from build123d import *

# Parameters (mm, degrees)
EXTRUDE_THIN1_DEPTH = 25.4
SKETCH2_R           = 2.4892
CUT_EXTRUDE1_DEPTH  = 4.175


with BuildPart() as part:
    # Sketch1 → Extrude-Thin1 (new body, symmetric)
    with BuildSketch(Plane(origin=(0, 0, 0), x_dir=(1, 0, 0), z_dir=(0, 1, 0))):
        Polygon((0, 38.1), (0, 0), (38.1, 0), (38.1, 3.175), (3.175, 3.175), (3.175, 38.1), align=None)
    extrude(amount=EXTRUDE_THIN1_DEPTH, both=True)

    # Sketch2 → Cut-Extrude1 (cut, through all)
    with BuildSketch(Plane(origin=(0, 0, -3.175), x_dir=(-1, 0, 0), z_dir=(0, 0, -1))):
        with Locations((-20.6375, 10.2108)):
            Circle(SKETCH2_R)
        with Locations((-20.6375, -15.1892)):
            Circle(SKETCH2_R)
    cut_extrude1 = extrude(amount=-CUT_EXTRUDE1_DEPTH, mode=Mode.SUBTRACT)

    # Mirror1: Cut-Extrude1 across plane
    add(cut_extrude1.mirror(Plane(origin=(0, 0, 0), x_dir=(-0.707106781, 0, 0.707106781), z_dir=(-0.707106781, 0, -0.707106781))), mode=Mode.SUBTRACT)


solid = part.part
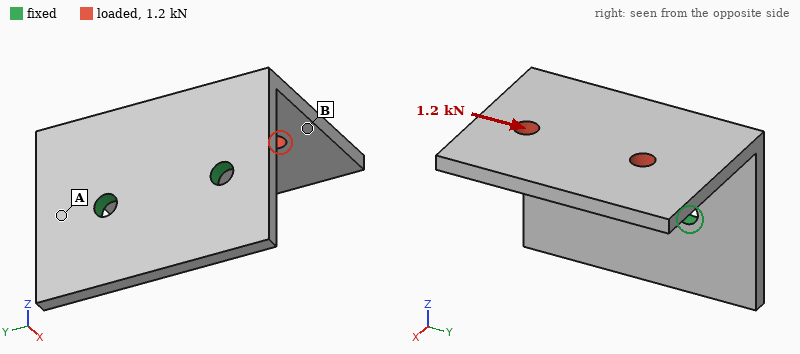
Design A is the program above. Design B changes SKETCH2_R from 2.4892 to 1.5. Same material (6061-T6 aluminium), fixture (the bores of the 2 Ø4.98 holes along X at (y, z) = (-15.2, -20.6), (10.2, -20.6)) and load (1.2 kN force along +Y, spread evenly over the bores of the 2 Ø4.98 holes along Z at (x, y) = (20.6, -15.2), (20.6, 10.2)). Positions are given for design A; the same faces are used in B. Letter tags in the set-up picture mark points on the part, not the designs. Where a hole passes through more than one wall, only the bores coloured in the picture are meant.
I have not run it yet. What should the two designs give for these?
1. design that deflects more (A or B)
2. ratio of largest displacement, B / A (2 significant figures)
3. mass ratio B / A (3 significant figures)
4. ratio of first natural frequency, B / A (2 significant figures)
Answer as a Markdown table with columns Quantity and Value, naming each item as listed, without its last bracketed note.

| Quantity | Value |
|---|---|
| design that deflects more | B |
| ratio of largest displacement, B / A | 1.2 |
| mass ratio B / A | 1.01 |
| ratio of first natural frequency, B / A | 0.94 |
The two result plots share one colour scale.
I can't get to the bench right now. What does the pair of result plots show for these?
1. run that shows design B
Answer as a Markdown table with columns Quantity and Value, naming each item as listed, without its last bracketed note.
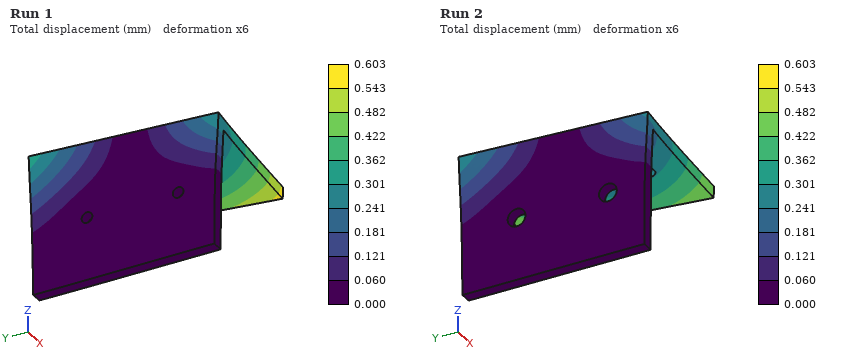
| Quantity | Value |
|---|---|
| run that shows design B | Run 1 |
